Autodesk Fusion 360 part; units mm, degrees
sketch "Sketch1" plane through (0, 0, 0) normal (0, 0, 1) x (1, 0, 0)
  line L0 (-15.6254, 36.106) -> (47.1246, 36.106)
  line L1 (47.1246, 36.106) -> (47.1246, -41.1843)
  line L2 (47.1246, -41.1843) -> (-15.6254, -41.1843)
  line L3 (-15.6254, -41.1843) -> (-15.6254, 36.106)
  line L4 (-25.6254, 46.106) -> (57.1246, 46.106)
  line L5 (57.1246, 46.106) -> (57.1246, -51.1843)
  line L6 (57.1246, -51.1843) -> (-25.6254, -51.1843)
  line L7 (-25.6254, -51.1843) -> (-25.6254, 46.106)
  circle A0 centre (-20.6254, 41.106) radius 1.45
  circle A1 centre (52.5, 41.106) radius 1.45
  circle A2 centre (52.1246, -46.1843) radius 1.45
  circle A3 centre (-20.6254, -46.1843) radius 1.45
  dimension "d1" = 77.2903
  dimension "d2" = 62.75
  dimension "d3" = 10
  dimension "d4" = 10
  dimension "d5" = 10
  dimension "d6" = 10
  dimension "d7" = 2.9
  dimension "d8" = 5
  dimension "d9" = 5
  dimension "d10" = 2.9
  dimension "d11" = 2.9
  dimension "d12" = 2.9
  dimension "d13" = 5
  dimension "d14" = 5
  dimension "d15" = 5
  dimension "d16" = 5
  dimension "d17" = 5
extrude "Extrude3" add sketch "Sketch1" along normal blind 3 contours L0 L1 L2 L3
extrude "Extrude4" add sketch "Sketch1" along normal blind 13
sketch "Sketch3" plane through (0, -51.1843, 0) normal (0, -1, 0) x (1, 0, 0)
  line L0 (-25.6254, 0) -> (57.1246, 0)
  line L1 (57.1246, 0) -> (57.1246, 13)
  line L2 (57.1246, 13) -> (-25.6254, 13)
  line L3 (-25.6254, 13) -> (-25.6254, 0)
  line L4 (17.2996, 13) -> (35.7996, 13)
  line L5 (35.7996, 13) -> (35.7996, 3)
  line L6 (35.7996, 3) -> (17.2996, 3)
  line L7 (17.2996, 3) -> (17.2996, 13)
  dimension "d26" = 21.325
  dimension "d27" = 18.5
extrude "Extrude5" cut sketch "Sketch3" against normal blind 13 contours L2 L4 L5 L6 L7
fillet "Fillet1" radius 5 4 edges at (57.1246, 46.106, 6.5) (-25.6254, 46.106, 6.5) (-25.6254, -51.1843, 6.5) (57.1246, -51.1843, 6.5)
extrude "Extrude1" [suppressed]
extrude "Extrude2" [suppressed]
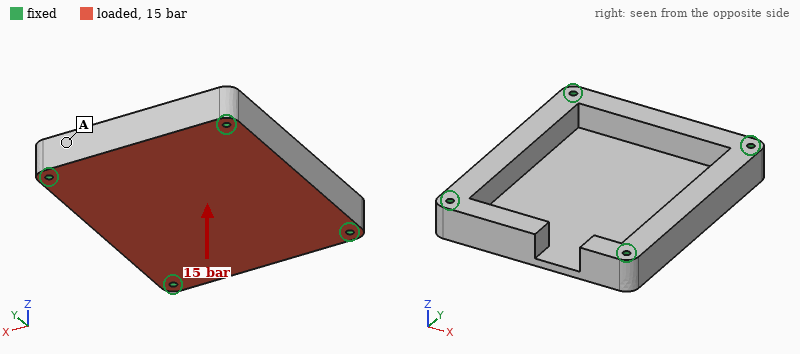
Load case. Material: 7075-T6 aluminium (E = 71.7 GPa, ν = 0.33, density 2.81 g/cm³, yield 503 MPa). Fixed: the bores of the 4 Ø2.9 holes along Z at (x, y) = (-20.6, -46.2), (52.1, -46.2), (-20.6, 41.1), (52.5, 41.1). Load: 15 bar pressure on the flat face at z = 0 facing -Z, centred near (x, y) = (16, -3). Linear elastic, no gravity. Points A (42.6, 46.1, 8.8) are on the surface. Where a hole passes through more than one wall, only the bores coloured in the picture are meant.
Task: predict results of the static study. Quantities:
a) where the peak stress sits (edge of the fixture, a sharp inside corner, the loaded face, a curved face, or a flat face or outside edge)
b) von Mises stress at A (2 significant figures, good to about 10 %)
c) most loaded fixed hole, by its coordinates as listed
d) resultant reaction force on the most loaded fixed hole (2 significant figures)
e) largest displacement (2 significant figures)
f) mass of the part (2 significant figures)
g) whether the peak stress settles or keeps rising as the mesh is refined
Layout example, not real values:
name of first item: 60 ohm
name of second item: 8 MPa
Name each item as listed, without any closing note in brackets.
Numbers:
where the peak stress sits: edge of the fixture
von Mises stress at A: 24 MPa
most loaded fixed hole, by its coordinates as listed: (-20.6, -46.2)
resultant reaction force on the most loaded fixed hole: 4.3 kN
largest displacement: 0.42 mm
mass of the part: 150 g
whether the peak stress settles or keeps rising as the mesh is refined: keeps rising
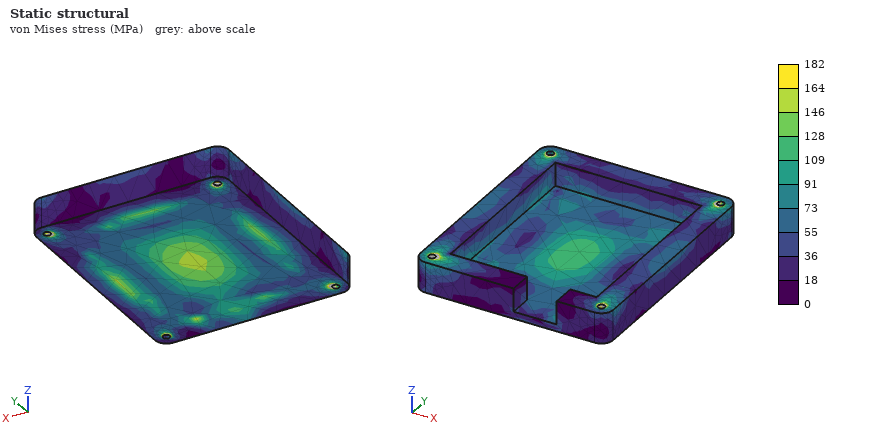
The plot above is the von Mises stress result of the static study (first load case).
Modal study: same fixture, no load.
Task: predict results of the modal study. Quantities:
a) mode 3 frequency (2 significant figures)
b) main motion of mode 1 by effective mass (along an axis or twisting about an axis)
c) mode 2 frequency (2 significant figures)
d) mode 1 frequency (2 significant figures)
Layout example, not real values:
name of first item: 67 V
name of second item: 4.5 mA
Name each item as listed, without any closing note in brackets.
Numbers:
mode 3 frequency: 6900 Hz
main motion of mode 1 by effective mass: along Z
mode 2 frequency: 6800 Hz
mode 1 frequency: 4100 Hz
